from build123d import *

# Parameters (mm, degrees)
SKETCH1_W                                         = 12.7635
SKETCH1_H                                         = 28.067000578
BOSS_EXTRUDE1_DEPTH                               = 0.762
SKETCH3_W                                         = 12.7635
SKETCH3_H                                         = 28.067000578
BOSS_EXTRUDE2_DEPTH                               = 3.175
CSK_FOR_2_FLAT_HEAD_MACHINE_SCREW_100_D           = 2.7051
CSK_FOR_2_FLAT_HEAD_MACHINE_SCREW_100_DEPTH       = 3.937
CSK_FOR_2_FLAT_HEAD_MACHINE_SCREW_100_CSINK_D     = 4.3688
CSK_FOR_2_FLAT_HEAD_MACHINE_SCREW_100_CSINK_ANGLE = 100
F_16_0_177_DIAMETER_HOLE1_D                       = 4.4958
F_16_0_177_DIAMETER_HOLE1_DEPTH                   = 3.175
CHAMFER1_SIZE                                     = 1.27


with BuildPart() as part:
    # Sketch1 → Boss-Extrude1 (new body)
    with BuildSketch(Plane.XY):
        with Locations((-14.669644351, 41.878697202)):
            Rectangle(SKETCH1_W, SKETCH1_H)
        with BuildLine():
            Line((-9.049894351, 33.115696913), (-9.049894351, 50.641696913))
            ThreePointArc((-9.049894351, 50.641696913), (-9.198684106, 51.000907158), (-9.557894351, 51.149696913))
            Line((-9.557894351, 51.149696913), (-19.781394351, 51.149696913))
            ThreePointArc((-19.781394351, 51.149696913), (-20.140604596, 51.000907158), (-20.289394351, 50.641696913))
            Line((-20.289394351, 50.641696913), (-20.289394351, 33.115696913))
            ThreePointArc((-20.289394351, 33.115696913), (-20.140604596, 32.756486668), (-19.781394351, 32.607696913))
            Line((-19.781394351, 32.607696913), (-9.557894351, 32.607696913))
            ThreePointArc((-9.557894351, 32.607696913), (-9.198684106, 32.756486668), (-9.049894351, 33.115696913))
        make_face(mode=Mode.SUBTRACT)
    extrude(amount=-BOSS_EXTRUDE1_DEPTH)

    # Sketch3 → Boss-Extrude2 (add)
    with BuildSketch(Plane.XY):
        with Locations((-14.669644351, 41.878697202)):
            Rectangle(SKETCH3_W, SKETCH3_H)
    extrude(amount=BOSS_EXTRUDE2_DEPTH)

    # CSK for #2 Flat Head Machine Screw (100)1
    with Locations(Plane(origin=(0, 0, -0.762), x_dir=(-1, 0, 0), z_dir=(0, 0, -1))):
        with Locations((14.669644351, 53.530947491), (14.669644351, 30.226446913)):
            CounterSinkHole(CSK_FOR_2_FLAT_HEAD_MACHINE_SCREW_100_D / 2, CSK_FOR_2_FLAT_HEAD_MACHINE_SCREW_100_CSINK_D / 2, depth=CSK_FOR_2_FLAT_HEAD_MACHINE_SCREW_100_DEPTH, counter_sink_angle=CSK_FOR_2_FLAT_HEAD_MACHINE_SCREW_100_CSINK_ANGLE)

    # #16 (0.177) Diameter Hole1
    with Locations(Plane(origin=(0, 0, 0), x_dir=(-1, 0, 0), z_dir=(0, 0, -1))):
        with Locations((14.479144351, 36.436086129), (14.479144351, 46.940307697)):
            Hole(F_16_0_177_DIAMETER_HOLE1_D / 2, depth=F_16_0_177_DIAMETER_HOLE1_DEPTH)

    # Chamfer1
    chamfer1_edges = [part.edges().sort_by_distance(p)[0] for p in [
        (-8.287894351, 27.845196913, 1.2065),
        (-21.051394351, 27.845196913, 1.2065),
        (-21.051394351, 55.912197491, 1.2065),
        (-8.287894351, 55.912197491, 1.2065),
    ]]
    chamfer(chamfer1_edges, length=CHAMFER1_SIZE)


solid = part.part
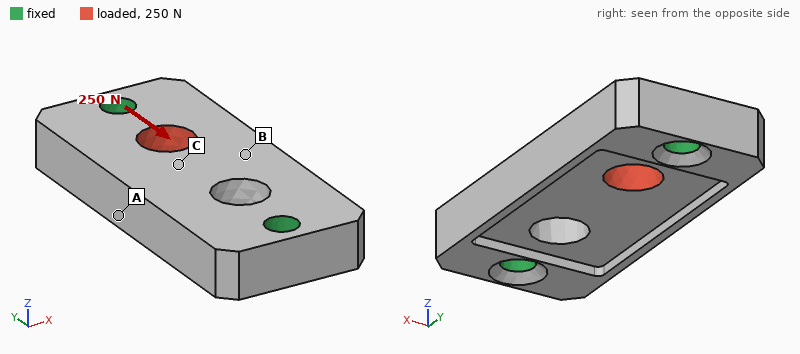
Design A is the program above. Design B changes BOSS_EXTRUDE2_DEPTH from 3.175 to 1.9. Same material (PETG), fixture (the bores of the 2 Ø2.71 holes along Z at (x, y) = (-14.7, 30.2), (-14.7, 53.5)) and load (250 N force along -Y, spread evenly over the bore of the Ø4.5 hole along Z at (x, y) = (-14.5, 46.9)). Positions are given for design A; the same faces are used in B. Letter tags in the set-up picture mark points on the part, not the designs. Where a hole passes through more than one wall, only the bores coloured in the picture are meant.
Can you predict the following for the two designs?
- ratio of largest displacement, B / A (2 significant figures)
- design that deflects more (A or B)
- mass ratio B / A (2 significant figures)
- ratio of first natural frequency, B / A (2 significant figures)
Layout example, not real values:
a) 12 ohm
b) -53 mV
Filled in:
a) 1.6
b) B
c) 0.63
d) 0.72
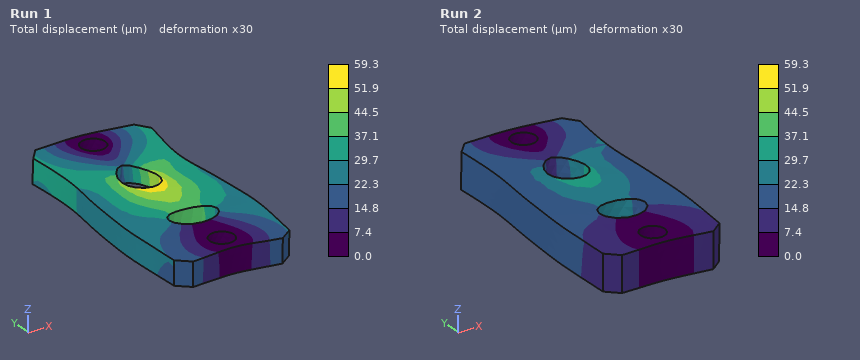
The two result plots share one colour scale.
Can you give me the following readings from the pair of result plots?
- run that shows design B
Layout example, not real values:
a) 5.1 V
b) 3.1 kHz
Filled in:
a) Run 1
